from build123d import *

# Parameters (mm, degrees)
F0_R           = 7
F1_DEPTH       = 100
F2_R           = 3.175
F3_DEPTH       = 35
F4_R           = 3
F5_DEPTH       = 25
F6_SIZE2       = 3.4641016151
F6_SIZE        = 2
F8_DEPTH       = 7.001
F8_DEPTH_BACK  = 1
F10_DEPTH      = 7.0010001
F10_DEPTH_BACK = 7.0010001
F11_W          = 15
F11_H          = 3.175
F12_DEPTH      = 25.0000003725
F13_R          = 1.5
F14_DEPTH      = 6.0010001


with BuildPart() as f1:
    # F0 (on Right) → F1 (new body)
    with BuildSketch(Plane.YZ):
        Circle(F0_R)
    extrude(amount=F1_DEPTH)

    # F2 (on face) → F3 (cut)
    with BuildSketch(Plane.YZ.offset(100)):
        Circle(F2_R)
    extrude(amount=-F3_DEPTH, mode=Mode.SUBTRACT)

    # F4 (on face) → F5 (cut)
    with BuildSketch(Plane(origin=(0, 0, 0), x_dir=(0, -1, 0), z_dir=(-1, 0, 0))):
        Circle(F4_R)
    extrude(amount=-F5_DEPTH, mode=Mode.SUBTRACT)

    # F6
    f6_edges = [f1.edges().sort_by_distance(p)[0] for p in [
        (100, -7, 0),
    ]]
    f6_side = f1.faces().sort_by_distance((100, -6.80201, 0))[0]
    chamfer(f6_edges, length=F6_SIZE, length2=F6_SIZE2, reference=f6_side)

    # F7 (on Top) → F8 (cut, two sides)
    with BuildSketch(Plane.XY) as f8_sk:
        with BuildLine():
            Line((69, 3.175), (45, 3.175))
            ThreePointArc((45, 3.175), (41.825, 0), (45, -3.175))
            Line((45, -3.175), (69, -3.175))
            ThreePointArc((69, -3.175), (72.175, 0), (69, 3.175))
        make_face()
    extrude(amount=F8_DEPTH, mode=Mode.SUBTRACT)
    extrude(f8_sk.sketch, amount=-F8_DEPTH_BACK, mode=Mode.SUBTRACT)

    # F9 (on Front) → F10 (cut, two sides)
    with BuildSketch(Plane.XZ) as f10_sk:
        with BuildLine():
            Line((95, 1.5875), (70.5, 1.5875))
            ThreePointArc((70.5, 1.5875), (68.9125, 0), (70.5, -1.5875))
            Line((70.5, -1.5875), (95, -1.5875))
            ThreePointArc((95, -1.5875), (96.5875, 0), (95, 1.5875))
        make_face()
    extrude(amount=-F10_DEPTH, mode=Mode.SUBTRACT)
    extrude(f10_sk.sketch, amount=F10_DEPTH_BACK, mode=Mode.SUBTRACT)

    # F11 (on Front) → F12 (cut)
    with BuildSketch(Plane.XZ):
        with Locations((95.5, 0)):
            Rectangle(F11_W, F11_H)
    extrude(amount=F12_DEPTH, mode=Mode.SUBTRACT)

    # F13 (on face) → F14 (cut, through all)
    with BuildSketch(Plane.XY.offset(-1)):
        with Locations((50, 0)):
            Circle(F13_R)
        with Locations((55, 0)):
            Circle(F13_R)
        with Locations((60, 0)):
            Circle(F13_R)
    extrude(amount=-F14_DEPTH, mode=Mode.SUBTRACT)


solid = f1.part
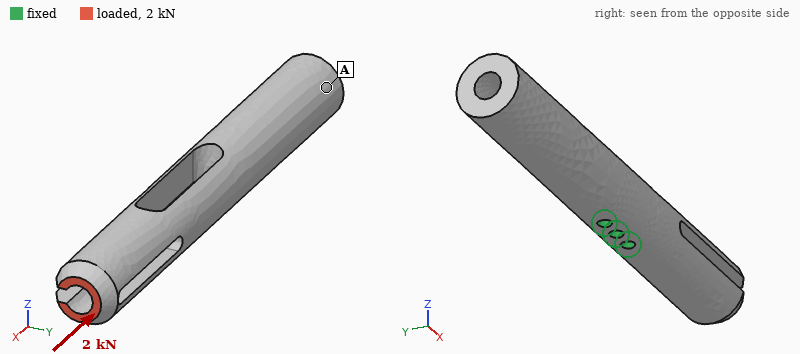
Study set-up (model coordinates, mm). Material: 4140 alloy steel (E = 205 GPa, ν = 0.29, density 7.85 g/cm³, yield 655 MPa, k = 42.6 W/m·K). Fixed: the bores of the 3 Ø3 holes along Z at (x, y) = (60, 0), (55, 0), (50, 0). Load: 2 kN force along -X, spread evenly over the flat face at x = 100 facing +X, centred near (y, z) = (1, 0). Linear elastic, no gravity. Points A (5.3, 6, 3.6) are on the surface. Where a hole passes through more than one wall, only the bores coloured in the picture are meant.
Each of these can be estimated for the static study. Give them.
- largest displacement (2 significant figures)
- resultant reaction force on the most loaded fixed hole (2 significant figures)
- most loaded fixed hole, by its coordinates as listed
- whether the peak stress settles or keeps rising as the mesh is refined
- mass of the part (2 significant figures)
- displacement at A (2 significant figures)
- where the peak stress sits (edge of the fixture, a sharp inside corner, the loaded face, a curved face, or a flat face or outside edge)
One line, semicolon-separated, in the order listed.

20 µm; 1.2 kN; (60, 0); keeps rising; 89 g; 4.8 µm; edge of the fixture
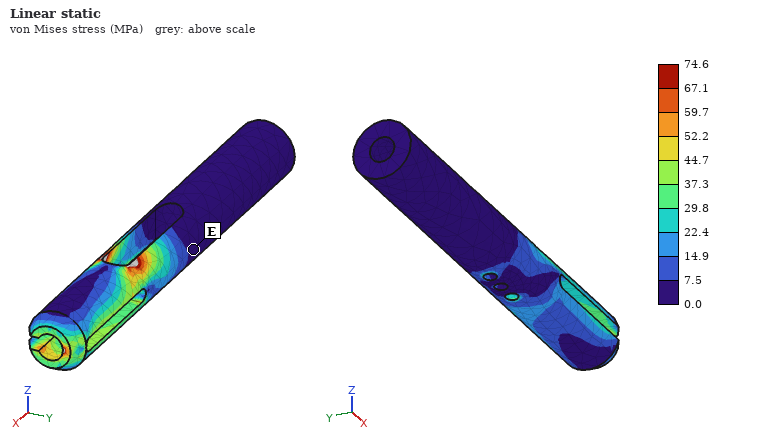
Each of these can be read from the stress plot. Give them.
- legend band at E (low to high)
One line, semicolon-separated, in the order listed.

0.0 to 7.5 MPa
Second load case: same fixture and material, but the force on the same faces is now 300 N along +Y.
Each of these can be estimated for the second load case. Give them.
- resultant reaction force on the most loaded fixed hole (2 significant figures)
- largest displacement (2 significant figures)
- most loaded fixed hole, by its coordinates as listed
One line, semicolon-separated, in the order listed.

1.1 kN; 39 µm; (60, 0)
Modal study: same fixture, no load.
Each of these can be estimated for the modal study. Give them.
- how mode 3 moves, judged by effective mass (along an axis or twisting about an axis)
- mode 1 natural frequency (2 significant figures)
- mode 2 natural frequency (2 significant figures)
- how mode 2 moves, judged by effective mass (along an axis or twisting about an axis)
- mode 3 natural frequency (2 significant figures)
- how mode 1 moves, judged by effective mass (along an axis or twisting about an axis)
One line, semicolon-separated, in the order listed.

along Z; 2900 Hz; 3100 Hz; along Y; 3500 Hz; along Z
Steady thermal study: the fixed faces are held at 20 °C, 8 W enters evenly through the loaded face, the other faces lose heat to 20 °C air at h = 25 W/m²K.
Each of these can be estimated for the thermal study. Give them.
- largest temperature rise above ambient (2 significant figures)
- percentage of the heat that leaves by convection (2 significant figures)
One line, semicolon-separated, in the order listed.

75 K; 29 %
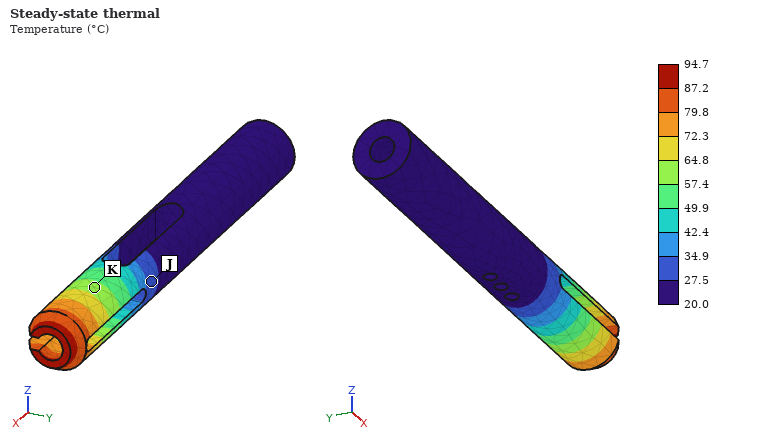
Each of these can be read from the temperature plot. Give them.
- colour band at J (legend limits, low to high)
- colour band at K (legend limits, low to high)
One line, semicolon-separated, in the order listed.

27.5 to 34.9 °C; 57.4 to 64.8 °C
